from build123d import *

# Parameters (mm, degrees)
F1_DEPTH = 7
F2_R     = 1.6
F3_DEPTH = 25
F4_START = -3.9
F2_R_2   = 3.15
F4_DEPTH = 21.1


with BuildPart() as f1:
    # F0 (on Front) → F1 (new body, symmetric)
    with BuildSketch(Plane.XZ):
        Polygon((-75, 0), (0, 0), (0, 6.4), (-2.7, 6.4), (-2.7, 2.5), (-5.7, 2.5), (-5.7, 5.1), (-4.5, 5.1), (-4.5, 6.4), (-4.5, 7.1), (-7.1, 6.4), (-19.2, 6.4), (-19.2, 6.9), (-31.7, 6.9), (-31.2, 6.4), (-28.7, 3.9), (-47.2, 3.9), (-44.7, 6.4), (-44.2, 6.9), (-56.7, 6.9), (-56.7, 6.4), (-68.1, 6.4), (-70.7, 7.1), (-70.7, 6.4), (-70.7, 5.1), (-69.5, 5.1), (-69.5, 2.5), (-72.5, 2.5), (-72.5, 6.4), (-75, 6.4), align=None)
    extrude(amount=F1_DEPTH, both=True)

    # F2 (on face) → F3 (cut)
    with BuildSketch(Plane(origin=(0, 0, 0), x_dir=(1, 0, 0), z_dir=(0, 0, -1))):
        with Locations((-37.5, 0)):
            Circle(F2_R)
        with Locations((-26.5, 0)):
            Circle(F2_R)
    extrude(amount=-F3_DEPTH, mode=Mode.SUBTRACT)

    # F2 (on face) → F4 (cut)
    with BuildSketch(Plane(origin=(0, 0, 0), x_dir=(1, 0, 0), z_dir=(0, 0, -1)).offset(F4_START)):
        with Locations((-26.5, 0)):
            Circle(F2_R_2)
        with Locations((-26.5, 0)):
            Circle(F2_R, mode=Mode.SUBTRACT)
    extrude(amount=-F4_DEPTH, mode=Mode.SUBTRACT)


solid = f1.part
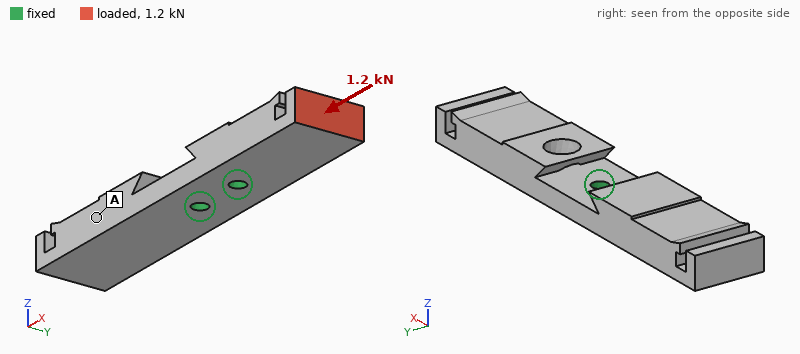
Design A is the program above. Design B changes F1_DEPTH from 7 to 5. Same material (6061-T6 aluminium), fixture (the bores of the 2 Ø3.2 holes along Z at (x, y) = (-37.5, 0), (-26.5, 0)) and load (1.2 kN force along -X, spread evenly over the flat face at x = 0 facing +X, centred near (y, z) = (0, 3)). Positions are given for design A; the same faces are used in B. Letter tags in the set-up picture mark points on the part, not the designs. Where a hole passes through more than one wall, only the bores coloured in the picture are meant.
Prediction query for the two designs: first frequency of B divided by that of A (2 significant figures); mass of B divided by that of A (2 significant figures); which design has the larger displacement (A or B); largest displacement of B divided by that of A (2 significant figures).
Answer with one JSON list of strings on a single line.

["1.0", "0.71", "B", "1.4"]
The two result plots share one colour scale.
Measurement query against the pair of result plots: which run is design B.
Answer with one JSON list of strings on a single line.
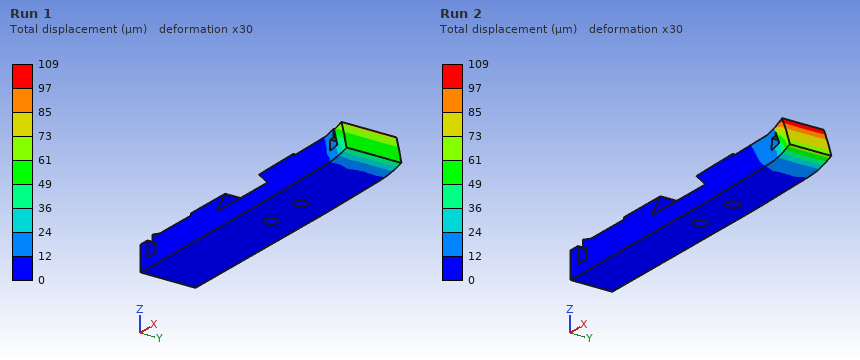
["Run 2"]
